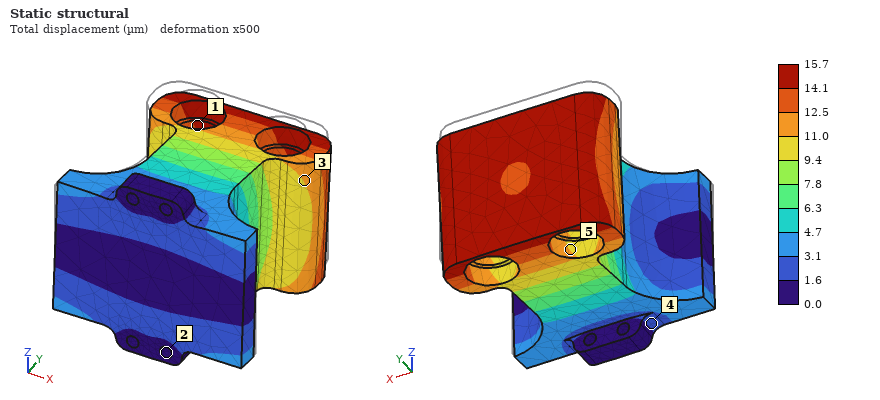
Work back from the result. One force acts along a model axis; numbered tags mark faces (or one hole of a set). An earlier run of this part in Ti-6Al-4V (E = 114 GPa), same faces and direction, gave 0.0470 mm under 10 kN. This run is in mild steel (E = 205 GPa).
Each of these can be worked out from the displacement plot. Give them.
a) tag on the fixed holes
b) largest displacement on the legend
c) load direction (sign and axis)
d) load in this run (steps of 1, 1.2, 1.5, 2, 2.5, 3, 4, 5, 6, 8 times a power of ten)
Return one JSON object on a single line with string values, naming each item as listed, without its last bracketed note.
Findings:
{"tag on the fixed holes": "2", "largest displacement on the legend": "15.7 µm", "load direction": "-Z", "load in this run": "6 kN"}
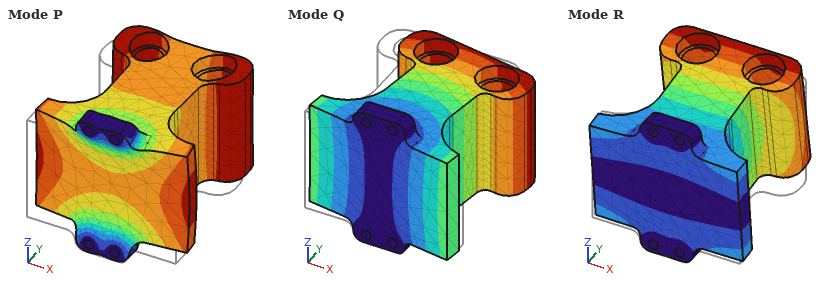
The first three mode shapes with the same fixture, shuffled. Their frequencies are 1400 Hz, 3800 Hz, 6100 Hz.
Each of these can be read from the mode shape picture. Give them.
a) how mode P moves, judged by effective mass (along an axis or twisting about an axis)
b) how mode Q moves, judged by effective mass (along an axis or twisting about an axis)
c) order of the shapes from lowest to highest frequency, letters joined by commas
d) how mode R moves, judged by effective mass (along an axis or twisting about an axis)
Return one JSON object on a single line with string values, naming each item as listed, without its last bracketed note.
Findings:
{"how mode P moves, judged by effective mass": "along Y", "how mode Q moves, judged by effective mass": "along X", "order of the shapes from lowest to highest frequency, letters joined by commas": "Q, R, P", "how mode R moves, judged by effective mass": "along Z"}
